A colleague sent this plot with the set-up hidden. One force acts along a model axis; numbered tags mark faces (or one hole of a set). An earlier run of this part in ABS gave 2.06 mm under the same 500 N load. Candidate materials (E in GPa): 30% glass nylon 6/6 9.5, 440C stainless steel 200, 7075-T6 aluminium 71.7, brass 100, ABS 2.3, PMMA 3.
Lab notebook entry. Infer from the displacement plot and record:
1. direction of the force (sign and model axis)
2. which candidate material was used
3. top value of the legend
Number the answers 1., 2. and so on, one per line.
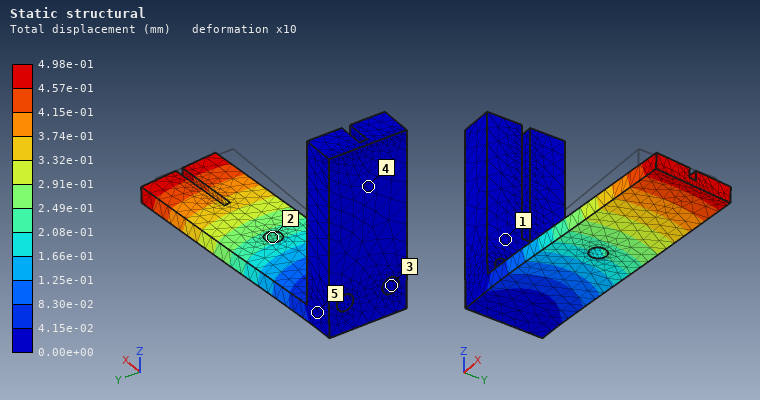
1. +Y
2. 30% glass nylon 6/6
3. 4.98e-01 mm
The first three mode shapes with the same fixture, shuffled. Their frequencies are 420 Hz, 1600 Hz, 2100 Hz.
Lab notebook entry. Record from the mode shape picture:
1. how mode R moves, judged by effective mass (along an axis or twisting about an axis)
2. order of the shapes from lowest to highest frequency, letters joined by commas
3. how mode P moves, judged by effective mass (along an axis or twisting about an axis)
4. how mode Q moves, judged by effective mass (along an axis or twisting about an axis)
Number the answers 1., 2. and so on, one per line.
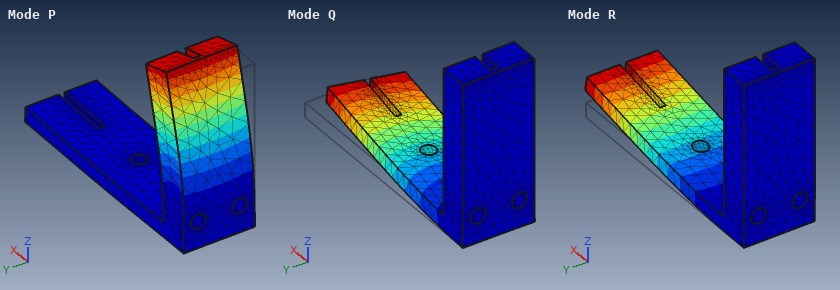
1. along Z
2. R, Q, P
3. along X
4. along Y
